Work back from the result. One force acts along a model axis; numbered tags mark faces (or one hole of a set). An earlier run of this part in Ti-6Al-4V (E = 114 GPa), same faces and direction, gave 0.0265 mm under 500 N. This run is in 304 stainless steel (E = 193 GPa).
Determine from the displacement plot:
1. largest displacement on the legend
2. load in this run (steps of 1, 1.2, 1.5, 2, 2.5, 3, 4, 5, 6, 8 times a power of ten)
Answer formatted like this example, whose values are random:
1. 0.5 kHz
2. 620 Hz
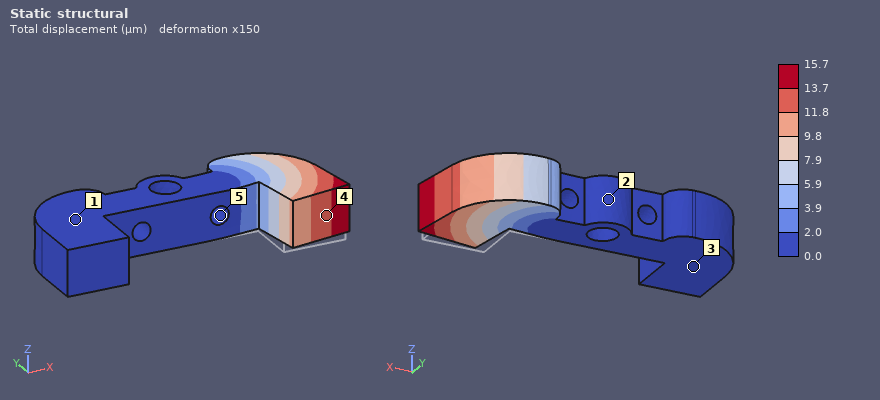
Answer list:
1. 15.7 µm
2. 500 N
